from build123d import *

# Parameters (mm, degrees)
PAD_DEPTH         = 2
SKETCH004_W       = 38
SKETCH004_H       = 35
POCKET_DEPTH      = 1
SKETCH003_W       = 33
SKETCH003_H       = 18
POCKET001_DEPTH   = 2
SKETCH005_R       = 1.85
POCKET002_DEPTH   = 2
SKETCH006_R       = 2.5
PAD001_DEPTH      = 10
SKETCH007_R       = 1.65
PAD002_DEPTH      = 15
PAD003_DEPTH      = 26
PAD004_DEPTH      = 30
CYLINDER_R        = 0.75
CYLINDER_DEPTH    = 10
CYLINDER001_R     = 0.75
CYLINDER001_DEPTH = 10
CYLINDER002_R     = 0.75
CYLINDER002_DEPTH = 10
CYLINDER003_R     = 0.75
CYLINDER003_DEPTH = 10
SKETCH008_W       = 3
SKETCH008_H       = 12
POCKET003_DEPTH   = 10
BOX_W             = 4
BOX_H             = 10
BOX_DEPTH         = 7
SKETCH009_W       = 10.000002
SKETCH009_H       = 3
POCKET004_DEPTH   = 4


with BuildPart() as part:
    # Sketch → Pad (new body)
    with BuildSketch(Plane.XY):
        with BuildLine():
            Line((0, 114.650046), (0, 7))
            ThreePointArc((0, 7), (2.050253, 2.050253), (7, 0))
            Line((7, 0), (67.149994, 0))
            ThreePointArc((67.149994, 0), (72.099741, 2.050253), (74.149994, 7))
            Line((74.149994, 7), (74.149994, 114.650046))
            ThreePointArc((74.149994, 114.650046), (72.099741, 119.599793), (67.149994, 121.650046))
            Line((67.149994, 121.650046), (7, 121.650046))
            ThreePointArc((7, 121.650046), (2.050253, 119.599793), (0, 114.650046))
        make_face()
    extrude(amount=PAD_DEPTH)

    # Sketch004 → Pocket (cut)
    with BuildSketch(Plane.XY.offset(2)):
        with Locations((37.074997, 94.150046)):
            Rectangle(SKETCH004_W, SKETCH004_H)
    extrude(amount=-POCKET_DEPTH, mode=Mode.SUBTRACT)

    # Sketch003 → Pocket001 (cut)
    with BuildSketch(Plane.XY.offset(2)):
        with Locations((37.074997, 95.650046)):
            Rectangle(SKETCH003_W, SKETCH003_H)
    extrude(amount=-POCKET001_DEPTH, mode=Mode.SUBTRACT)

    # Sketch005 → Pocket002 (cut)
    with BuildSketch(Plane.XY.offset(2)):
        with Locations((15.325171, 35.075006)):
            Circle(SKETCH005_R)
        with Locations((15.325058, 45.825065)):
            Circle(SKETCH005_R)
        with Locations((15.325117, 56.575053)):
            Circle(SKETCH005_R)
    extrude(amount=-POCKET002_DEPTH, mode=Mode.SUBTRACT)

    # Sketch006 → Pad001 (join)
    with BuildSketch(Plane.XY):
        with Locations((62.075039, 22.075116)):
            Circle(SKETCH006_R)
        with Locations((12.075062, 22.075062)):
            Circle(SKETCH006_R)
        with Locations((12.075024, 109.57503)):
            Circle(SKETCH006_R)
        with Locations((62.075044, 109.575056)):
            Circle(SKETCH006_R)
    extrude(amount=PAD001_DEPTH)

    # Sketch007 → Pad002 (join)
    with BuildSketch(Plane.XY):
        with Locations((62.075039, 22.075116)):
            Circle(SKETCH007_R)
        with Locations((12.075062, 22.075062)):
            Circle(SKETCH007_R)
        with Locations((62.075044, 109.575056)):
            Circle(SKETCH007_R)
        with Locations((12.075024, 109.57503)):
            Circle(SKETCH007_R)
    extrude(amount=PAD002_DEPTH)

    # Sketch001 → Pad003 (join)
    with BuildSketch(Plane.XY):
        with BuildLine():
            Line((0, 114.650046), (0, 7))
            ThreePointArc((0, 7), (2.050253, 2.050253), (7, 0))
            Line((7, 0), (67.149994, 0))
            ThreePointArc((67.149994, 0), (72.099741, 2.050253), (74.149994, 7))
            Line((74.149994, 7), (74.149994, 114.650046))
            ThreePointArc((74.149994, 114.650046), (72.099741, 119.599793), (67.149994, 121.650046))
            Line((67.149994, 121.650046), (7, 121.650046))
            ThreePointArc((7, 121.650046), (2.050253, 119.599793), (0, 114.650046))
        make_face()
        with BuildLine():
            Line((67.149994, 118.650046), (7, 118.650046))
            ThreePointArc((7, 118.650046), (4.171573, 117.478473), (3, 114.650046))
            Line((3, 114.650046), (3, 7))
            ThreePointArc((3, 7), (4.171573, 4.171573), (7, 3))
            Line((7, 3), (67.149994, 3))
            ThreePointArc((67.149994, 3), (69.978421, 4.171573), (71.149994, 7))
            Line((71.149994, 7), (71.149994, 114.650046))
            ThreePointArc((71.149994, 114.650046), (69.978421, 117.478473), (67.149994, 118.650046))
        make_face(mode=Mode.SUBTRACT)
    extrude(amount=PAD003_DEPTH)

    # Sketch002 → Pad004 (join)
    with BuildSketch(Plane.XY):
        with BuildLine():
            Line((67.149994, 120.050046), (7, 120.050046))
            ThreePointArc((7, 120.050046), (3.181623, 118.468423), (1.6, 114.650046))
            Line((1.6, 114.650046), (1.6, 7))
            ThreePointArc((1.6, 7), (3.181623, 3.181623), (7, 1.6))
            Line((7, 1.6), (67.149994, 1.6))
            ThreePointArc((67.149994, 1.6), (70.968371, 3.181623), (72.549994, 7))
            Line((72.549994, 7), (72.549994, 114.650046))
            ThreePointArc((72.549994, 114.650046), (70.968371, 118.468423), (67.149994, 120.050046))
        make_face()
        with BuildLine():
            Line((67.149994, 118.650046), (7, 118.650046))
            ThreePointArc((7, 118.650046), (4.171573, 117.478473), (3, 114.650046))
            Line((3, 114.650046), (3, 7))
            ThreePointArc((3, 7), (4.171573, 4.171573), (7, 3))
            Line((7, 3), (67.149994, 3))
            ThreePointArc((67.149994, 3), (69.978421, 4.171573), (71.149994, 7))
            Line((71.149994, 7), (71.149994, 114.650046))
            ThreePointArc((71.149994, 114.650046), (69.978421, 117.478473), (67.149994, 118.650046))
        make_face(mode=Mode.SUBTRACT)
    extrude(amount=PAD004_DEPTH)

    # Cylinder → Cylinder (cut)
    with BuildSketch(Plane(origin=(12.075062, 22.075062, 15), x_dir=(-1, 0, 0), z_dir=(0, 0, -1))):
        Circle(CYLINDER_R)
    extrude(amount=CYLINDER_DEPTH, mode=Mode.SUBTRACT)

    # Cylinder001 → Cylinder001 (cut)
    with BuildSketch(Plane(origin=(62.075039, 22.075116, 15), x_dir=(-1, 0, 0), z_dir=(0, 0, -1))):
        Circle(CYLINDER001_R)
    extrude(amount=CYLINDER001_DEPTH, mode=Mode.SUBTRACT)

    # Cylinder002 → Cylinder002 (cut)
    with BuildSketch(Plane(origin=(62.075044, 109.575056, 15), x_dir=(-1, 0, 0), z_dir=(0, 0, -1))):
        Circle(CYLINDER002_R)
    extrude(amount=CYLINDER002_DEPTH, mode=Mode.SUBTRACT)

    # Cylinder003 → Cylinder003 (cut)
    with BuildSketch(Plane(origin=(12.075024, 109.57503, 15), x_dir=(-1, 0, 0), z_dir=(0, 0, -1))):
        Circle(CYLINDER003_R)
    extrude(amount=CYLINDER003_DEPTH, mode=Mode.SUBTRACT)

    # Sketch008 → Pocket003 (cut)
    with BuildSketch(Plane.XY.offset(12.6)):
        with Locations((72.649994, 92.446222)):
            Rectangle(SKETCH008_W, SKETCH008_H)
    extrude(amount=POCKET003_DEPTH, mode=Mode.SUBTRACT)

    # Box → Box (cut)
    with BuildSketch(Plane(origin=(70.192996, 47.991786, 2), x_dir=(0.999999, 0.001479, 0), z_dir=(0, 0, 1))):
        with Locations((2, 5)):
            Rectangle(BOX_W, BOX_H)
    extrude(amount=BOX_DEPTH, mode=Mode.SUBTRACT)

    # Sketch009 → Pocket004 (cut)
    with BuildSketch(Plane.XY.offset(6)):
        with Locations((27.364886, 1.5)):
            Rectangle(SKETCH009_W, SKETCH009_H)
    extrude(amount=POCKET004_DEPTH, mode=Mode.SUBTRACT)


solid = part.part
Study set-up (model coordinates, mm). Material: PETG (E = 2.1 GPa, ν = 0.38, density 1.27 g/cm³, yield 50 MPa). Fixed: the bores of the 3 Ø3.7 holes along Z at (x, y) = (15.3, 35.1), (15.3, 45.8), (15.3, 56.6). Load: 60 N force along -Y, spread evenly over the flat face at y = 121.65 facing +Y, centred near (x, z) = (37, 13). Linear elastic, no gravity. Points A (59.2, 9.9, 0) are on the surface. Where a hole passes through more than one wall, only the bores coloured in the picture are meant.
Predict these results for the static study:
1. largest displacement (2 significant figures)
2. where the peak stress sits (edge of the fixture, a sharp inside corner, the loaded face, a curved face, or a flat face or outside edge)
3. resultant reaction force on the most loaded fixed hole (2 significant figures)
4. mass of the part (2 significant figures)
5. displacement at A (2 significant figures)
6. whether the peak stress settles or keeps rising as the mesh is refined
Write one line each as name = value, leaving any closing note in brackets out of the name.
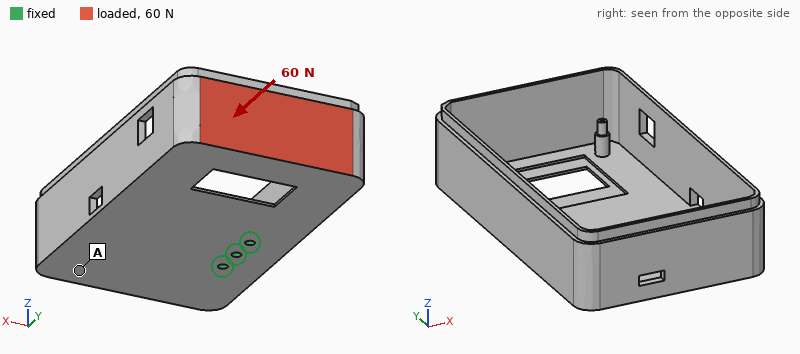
largest displacement = 1.7 mm
where the peak stress sits = edge of the fixture
resultant reaction force on the most loaded fixed hole = 64 N
mass of the part = 57 g
displacement at A = 0.60 mm
whether the peak stress settles or keeps rising as the mesh is refined = keeps rising
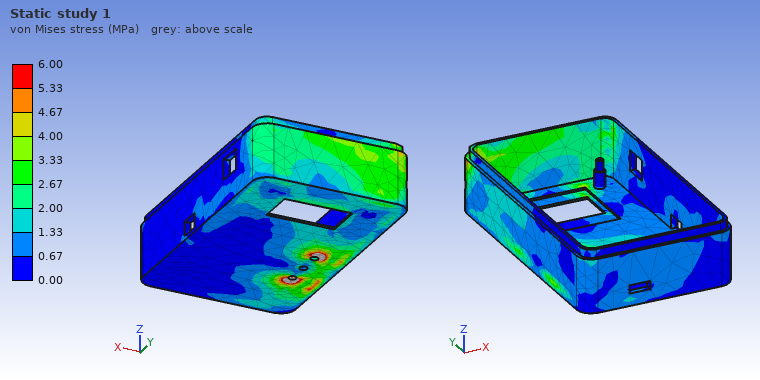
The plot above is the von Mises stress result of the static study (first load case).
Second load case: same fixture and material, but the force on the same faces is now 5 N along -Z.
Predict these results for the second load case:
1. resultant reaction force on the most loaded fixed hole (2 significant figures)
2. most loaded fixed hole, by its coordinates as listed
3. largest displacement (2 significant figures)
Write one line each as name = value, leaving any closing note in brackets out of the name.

resultant reaction force on the most loaded fixed hole = 16 N
most loaded fixed hole, by its coordinates as listed = (15.3, 56.6)
largest displacement = 1.6 mm
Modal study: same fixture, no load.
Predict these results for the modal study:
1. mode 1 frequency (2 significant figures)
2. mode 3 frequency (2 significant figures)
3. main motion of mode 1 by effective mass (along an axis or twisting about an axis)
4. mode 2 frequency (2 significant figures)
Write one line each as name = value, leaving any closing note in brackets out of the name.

mode 1 frequency = 60 Hz
mode 3 frequency = 190 Hz
main motion of mode 1 by effective mass = along Z
mode 2 frequency = 100 Hz
